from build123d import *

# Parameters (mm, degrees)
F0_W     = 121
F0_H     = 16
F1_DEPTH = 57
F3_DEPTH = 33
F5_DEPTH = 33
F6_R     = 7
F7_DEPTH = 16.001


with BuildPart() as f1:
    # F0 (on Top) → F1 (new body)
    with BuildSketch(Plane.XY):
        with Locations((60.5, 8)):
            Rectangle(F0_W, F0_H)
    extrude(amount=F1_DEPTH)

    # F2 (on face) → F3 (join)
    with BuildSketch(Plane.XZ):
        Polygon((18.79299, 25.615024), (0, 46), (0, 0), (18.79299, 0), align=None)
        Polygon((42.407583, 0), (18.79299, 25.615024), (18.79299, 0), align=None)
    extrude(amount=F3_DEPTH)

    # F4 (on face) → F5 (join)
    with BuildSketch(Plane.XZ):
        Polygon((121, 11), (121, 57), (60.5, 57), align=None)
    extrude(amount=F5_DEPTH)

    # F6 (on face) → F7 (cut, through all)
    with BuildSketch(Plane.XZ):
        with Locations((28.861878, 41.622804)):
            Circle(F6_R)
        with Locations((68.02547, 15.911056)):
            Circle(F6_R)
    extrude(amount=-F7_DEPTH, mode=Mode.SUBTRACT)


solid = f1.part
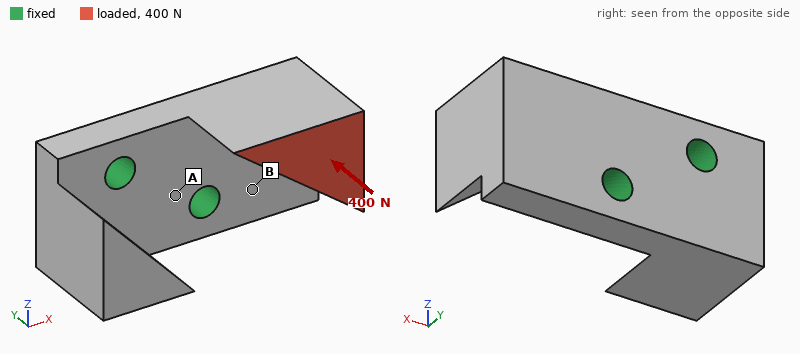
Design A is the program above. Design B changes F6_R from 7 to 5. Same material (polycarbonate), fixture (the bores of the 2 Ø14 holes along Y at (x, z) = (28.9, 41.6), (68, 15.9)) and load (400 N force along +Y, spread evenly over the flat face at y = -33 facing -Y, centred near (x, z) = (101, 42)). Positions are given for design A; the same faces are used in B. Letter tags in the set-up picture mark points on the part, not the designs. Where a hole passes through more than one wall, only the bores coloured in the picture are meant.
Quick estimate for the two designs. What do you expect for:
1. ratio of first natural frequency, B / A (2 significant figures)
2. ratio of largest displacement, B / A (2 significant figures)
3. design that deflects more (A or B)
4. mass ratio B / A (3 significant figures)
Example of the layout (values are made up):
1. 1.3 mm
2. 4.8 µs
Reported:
1. 0.92
2. 1.2
3. B
4. 1.01
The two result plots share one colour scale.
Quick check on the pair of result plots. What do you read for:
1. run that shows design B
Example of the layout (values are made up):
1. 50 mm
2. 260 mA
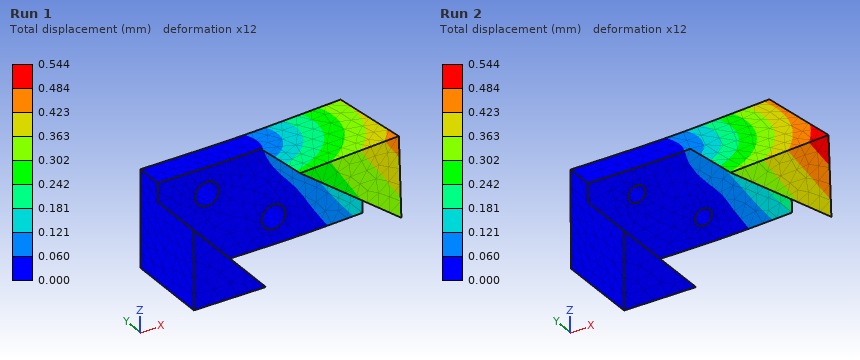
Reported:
1. Run 2
